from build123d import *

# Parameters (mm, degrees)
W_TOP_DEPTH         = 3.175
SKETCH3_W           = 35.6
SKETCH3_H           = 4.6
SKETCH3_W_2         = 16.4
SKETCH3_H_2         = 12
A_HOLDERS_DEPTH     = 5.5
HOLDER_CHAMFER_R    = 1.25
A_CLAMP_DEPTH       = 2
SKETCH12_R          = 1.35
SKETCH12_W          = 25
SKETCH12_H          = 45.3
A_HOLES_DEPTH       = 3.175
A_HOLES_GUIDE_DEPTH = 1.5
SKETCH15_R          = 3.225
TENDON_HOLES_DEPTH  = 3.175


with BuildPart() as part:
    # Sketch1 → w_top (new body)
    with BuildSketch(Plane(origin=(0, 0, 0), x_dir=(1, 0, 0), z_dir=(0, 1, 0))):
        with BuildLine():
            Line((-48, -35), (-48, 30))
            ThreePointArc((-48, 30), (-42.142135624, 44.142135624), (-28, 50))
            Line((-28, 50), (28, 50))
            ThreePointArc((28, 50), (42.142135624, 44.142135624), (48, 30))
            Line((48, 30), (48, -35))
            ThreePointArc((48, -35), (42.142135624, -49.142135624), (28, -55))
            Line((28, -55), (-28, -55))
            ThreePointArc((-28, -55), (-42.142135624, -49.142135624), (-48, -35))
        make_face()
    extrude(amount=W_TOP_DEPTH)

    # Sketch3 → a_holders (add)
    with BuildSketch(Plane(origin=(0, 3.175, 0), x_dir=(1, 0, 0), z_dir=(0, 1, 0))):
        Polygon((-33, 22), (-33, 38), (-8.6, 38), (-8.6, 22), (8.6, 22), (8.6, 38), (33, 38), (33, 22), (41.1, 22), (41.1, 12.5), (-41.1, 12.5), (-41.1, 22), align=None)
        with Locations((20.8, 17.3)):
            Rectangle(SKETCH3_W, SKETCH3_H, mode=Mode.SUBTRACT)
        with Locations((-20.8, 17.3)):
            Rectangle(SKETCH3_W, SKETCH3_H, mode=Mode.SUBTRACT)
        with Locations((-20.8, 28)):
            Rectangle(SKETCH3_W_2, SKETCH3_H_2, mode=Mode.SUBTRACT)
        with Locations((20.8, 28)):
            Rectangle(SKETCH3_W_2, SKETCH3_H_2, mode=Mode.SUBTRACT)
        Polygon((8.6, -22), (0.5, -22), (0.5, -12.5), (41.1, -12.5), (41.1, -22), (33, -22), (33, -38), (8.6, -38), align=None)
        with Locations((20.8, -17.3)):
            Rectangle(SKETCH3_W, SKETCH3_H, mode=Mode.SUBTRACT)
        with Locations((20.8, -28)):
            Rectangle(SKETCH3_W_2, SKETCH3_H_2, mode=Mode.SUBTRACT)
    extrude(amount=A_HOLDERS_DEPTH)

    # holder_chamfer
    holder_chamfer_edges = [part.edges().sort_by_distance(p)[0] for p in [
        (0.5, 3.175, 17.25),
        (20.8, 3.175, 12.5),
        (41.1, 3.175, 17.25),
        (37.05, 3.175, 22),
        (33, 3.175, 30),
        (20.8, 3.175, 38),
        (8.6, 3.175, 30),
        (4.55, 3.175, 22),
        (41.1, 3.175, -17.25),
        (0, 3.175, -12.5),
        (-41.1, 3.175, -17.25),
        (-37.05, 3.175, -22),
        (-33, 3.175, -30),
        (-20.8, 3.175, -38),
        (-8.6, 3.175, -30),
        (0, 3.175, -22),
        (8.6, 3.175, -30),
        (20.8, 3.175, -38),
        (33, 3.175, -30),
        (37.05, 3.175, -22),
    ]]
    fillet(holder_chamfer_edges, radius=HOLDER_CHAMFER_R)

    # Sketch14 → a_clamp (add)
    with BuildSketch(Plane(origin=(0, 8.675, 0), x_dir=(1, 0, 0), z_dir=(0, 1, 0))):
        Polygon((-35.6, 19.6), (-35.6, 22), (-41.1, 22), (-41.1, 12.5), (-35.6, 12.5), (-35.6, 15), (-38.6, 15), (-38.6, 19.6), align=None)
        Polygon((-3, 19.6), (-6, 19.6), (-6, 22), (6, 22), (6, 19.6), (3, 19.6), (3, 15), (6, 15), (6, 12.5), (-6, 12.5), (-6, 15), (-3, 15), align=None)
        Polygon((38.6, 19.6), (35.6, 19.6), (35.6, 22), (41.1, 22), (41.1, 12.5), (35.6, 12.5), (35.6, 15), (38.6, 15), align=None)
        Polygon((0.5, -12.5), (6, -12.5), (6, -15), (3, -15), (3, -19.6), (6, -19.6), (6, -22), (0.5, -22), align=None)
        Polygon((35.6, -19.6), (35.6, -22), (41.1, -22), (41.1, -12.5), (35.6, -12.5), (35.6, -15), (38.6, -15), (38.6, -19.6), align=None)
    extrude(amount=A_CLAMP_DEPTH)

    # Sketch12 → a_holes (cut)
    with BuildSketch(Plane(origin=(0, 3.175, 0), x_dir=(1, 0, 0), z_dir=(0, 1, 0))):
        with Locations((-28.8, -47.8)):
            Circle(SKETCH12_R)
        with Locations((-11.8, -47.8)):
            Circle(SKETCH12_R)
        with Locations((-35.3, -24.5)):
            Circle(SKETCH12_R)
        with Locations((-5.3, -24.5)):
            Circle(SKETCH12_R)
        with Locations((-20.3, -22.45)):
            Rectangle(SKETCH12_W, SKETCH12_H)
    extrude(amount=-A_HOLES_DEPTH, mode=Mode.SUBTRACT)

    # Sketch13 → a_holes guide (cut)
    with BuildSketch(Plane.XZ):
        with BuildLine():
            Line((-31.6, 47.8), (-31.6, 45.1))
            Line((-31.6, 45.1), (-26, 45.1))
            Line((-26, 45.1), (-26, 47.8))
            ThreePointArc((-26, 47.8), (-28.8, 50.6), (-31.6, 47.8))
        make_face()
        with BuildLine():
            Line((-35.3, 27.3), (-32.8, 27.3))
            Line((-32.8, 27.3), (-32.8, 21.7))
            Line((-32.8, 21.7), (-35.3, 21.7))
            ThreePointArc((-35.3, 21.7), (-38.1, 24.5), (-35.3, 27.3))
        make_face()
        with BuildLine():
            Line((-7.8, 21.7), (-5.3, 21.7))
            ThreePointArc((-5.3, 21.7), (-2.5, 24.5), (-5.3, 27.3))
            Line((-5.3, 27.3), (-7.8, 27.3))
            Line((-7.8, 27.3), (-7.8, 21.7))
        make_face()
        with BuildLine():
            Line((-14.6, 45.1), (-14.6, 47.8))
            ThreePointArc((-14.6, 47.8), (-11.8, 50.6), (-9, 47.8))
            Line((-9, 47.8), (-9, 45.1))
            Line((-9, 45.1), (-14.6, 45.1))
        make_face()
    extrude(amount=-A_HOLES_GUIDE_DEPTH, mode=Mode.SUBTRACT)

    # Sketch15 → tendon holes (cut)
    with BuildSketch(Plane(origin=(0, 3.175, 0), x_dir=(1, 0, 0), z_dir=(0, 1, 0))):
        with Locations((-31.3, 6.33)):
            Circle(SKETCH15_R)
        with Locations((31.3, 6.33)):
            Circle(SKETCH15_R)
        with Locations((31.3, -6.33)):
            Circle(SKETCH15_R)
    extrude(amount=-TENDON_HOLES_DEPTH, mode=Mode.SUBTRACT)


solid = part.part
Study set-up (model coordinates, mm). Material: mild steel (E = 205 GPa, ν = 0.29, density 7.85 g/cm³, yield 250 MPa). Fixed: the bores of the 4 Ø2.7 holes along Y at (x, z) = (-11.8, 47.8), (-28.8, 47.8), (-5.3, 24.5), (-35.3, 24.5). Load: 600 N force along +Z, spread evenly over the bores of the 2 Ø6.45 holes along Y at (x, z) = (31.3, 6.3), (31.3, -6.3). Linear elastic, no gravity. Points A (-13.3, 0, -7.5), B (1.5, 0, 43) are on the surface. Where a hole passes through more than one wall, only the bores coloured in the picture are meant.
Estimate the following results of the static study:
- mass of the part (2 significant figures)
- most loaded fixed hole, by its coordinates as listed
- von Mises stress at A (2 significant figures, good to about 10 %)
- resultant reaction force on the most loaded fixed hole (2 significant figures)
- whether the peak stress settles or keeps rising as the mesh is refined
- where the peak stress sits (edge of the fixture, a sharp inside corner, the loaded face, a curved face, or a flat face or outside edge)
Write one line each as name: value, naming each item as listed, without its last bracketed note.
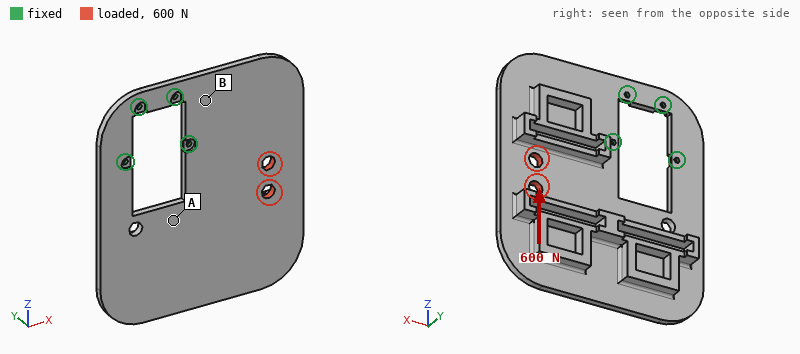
mass of the part: 270 g
most loaded fixed hole, by its coordinates as listed: (-5.3, 24.5)
von Mises stress at A: 5.2 MPa
resultant reaction force on the most loaded fixed hole: 810 N
whether the peak stress settles or keeps rising as the mesh is refined: keeps rising
where the peak stress sits: edge of the fixture
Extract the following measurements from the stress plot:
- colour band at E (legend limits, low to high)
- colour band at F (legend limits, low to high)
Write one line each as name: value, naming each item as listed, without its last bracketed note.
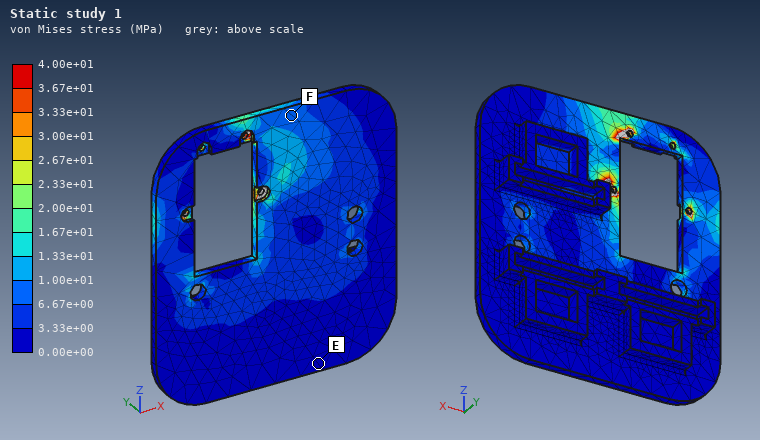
colour band at E: 0.00e+00 to 3.33e+00 MPa
colour band at F: 6.67e+00 to 1.00e+01 MPa
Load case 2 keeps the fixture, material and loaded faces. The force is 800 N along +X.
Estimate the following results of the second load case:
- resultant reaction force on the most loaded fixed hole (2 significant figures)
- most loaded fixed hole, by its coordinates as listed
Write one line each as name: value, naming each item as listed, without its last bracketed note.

resultant reaction force on the most loaded fixed hole: 980 N
most loaded fixed hole, by its coordinates as listed: (-5.3, 24.5)
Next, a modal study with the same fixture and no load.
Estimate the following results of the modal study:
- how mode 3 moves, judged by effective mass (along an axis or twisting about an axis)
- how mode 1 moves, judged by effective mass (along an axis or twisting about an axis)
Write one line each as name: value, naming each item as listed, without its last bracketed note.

how mode 3 moves, judged by effective mass: along Y
how mode 1 moves, judged by effective mass: along Y
